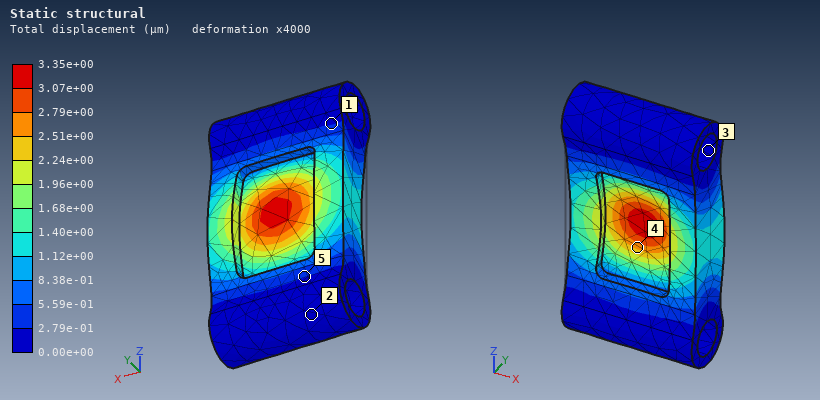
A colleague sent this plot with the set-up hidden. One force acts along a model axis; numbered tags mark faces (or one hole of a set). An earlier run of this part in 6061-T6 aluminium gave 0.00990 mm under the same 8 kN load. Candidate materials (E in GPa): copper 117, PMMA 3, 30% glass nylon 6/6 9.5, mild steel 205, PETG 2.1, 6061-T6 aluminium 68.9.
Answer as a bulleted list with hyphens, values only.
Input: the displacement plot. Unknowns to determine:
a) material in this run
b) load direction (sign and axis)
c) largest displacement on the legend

- mild steel
- +Y
- 3.35e+00 µm
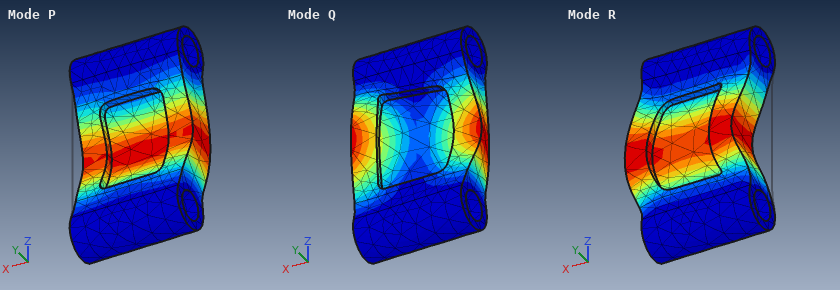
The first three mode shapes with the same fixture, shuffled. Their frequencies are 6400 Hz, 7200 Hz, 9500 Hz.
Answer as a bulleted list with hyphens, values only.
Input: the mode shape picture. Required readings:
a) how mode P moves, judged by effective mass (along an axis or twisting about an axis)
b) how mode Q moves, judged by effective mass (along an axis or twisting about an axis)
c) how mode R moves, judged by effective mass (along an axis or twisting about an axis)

- along Y
- twisting about Z
- along X
